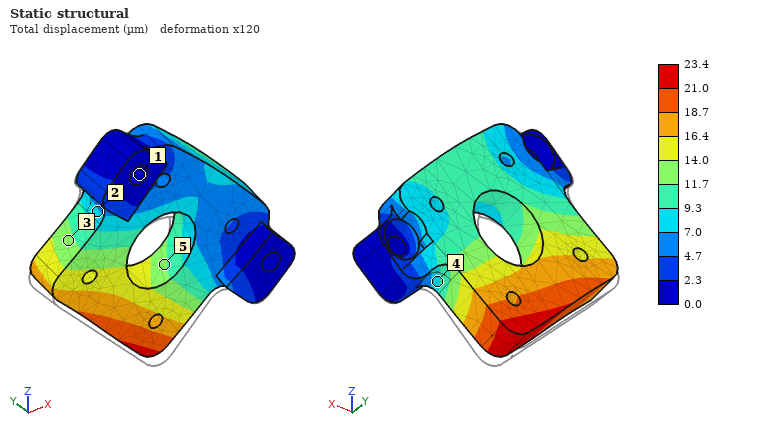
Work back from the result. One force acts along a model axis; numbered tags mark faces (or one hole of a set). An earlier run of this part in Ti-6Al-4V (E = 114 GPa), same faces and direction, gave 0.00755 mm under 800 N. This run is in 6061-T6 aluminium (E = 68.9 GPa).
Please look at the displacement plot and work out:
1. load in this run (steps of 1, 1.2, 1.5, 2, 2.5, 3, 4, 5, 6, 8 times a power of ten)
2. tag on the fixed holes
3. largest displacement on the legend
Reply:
1.5 kN
1
23.4 µm
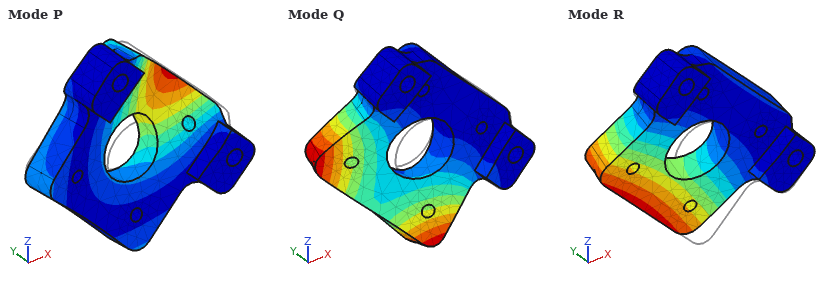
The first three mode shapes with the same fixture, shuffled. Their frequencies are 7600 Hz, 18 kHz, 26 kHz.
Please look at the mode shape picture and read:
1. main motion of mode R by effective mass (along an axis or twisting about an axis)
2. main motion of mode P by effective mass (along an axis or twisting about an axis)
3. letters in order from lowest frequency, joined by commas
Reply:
along Y
along Y
R, Q, P
